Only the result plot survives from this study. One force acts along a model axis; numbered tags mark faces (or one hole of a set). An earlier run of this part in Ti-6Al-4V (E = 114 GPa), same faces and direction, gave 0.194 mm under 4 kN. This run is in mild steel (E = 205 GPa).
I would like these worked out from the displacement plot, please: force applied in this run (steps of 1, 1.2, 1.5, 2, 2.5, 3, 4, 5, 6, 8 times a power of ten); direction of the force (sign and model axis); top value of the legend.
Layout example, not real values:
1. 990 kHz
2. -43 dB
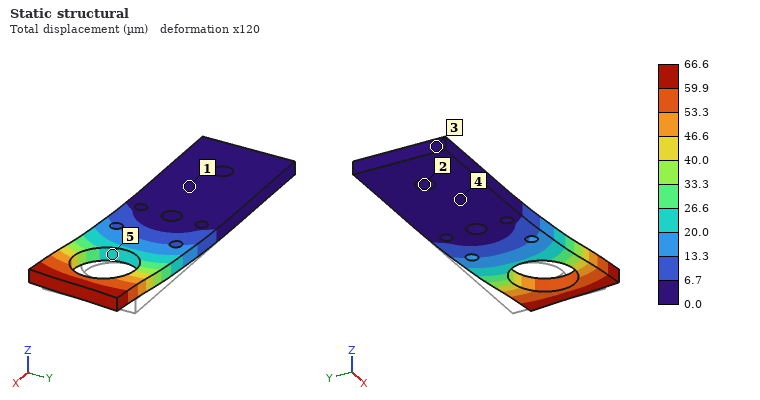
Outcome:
1. 2.5 kN
2. -Y
3. 66.6 µm
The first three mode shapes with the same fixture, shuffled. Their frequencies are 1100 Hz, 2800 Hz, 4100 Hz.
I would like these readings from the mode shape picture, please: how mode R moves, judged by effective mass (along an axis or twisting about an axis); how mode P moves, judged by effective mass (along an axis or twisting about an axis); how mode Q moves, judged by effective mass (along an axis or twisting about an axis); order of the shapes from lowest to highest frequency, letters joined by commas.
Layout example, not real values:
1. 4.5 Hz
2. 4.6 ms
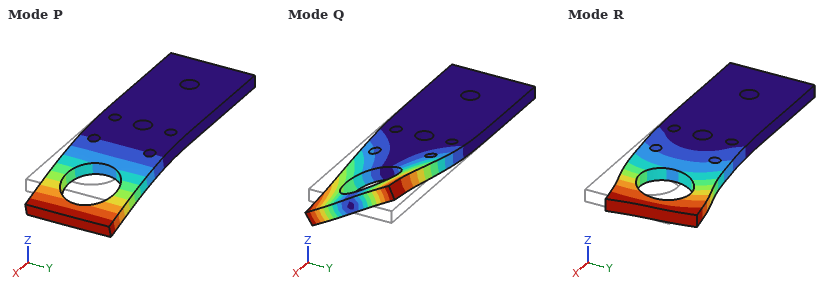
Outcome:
1. along Y
2. along Z
3. twisting about X
4. P, Q, R
